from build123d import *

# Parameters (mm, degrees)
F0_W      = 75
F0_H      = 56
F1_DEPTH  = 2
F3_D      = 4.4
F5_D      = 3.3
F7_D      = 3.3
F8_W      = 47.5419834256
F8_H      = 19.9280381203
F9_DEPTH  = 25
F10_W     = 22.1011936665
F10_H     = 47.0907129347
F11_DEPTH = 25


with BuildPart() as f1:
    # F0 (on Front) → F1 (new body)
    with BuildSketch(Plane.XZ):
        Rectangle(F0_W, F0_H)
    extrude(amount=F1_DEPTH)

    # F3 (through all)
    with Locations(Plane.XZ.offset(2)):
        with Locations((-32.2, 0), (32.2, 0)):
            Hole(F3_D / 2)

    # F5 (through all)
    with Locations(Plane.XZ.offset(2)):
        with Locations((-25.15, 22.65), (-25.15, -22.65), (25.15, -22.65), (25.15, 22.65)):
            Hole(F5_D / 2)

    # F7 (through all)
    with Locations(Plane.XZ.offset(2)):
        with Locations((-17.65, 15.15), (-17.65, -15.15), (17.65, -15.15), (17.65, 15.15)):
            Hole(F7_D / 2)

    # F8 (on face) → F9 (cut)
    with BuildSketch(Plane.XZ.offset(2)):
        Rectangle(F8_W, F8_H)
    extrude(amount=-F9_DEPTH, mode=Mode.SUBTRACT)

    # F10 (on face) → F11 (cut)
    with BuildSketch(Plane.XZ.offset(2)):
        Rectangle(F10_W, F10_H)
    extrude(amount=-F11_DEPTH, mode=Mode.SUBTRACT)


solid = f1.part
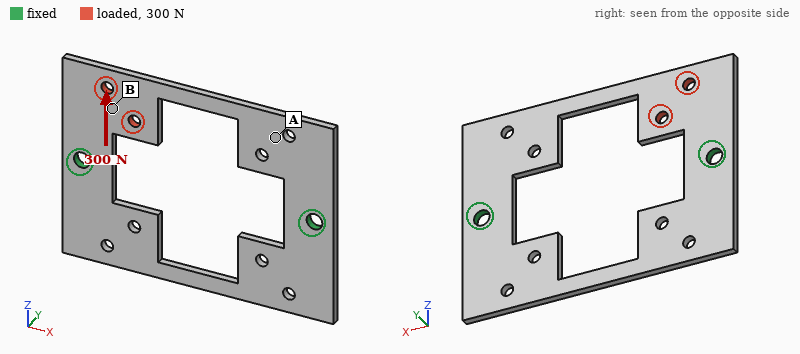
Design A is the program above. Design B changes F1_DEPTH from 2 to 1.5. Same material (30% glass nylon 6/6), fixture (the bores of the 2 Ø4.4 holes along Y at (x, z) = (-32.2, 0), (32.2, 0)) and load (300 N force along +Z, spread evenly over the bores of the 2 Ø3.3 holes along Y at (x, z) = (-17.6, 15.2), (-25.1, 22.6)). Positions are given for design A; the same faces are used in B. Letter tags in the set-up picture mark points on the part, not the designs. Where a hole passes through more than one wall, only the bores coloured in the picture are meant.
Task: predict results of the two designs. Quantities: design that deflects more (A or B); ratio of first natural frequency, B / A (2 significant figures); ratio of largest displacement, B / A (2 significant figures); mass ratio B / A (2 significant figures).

B
0.76
1.3
0.75
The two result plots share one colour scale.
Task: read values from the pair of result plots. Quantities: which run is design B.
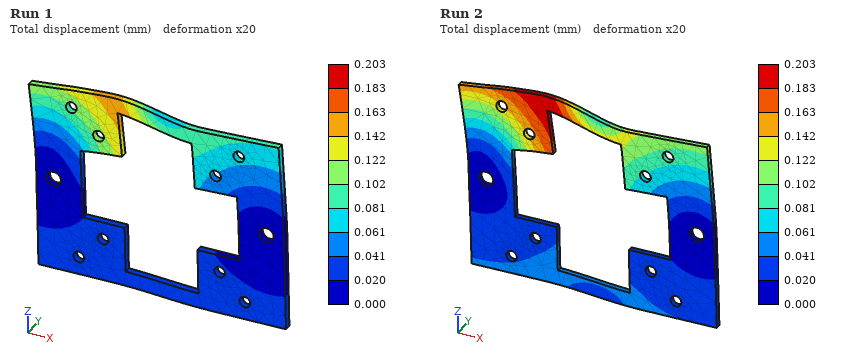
Run 2
